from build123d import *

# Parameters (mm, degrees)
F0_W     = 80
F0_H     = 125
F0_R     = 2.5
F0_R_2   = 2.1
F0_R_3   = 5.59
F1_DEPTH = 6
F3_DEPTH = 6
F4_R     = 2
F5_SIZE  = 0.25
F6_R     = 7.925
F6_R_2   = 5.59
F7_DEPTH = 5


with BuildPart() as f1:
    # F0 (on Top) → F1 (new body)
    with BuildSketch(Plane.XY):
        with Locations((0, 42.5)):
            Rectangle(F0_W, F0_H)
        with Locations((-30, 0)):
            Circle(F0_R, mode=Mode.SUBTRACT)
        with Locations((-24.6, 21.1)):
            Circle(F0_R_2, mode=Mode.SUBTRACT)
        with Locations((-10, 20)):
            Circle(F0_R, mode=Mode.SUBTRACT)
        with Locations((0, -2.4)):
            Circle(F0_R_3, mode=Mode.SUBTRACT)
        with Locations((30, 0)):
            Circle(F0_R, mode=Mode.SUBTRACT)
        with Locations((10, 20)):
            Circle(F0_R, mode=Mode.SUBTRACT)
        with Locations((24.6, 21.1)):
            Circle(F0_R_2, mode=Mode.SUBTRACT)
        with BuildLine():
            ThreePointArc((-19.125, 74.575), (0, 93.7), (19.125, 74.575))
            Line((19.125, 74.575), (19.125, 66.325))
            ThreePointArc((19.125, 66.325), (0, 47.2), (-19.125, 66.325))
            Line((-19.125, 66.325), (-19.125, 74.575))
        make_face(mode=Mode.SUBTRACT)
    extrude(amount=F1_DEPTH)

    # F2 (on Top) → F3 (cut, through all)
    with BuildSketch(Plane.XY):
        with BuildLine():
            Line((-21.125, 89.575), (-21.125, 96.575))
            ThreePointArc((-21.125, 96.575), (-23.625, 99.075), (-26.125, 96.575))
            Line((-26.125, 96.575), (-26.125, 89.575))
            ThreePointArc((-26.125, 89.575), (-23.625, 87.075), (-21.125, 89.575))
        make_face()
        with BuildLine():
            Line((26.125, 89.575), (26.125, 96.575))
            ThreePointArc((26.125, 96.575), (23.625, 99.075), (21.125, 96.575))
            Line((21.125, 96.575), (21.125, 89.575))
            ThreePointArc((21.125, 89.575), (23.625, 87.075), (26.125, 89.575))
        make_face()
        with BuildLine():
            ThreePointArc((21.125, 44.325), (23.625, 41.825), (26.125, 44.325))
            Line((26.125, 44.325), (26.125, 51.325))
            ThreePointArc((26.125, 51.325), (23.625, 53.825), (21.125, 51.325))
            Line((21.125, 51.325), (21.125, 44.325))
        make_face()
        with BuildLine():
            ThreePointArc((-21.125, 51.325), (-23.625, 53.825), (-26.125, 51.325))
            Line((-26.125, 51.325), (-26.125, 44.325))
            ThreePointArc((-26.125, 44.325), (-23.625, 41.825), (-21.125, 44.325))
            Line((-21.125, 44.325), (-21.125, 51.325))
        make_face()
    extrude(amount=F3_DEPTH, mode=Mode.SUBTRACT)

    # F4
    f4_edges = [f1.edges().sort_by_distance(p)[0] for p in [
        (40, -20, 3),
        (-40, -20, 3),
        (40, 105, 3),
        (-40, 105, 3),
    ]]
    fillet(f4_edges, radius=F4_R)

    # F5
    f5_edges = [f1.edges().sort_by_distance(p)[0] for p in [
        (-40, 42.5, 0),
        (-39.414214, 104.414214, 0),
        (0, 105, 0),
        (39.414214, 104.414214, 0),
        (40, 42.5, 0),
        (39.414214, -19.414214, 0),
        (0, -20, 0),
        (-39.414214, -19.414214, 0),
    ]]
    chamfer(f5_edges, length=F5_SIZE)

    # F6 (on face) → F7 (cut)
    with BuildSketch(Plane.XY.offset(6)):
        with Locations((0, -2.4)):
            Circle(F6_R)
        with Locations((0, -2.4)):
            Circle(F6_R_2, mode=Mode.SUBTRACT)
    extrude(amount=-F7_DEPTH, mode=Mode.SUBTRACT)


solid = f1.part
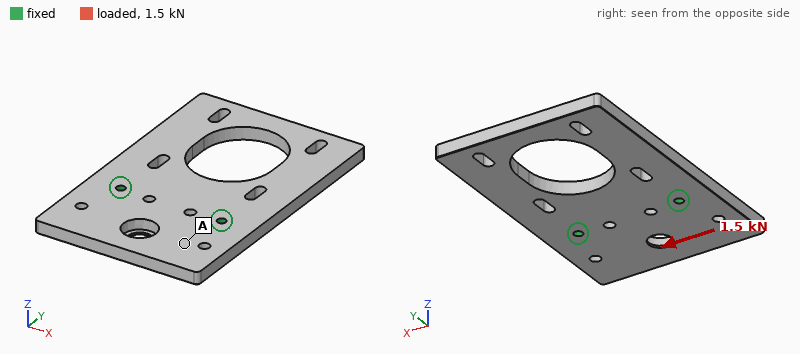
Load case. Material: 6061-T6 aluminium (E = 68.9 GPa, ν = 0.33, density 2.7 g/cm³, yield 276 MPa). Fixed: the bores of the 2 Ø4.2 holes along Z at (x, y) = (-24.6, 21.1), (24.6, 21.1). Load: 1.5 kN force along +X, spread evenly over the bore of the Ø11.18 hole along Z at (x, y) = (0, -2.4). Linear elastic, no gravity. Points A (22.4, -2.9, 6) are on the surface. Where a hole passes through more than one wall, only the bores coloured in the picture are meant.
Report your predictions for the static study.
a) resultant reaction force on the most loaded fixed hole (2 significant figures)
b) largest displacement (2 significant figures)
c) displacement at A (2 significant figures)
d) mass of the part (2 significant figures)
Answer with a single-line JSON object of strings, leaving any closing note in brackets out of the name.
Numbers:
{"resultant reaction force on the most loaded fixed hole": "1.0 kN", "largest displacement": "15 µm", "displacement at A": "7.2 µm", "mass of the part": "130 g"}
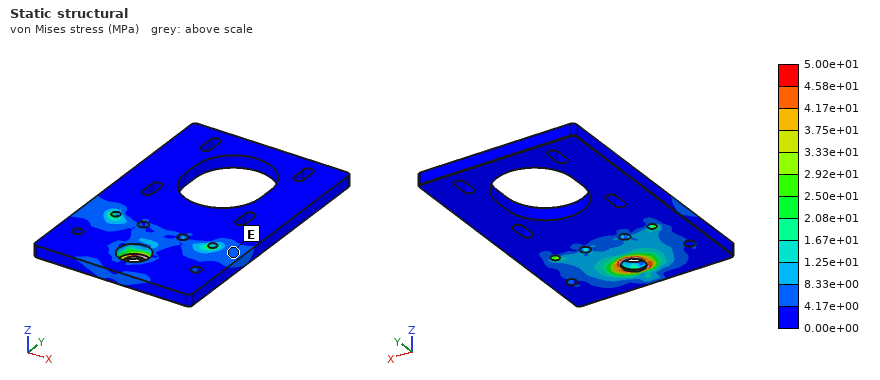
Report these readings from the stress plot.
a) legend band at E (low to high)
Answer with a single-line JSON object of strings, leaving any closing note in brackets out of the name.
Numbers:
{"legend band at E": "4.17e+00 to 8.33e+00 MPa"}
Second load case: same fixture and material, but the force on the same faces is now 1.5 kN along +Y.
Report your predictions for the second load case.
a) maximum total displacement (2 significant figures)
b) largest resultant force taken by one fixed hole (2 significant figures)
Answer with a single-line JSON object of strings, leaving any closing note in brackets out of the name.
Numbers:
{"maximum total displacement": "38 µm", "largest resultant force taken by one fixed hole": "780 N"}
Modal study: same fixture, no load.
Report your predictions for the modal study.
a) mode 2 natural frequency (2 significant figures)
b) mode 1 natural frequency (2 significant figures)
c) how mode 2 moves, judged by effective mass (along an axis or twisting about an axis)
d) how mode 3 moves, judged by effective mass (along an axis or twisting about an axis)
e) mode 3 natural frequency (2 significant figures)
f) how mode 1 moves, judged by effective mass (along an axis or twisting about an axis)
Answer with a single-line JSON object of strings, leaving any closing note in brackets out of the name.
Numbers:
{"mode 2 natural frequency": "1400 Hz", "mode 1 natural frequency": "660 Hz", "how mode 2 moves, judged by effective mass": "twisting about Y", "how mode 3 moves, judged by effective mass": "along Z", "mode 3 natural frequency": "2500 Hz", "how mode 1 moves, judged by effective mass": "along Z"}
